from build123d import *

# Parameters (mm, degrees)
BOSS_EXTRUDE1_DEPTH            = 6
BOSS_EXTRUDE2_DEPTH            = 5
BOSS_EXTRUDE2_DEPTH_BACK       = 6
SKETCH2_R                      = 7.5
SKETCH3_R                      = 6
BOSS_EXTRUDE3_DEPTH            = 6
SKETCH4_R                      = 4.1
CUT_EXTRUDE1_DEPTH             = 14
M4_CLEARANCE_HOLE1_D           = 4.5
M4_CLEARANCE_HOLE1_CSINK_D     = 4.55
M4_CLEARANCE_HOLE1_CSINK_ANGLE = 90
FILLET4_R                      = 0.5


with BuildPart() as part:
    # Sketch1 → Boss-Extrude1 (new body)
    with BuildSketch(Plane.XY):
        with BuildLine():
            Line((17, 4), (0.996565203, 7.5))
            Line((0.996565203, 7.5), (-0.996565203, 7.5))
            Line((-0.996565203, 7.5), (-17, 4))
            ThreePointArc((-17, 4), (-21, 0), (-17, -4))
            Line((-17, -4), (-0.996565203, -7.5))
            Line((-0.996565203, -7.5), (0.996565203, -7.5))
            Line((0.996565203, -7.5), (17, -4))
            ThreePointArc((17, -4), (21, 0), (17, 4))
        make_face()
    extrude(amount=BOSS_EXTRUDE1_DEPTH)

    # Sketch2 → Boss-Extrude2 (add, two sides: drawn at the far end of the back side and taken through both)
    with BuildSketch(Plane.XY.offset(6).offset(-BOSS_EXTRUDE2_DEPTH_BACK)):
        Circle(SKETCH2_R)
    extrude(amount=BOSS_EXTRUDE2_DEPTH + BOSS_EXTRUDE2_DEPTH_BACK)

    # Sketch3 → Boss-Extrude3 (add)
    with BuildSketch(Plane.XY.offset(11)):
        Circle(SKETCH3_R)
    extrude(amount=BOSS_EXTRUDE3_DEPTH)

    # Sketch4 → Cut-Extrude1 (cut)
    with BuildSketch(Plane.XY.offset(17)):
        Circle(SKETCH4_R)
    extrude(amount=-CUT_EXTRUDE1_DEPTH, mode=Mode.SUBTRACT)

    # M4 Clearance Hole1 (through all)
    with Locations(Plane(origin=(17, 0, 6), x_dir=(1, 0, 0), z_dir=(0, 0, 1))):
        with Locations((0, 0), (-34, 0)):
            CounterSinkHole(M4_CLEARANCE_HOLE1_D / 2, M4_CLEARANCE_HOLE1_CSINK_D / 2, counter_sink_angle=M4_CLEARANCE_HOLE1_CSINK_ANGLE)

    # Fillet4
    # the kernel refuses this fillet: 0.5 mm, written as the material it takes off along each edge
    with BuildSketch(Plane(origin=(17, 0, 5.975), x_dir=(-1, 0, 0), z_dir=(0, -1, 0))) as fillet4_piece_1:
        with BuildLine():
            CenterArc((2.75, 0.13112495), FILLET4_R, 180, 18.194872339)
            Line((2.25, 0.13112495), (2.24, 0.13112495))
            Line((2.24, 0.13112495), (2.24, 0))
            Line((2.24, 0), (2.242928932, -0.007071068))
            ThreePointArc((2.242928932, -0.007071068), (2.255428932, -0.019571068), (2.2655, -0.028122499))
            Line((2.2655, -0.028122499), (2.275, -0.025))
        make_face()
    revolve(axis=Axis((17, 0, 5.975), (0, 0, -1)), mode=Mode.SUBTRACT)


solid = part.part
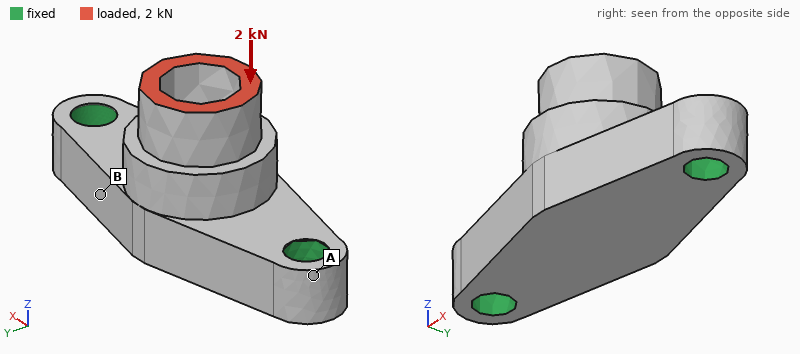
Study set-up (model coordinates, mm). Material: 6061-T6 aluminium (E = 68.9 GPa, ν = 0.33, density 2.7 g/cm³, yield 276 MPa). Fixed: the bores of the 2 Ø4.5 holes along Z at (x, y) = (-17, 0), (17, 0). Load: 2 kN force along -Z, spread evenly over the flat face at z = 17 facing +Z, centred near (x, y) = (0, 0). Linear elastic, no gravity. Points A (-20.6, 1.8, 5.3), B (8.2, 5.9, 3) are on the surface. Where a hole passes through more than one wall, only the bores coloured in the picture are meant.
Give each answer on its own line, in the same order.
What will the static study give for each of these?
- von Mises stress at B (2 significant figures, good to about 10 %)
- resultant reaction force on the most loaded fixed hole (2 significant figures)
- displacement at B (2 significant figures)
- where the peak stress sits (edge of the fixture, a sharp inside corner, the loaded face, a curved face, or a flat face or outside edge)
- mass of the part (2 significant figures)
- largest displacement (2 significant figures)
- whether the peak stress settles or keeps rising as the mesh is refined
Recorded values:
38 MPa
1.0 kN
14 µm
edge of the fixture
9.0 g
23 µm
keeps rising
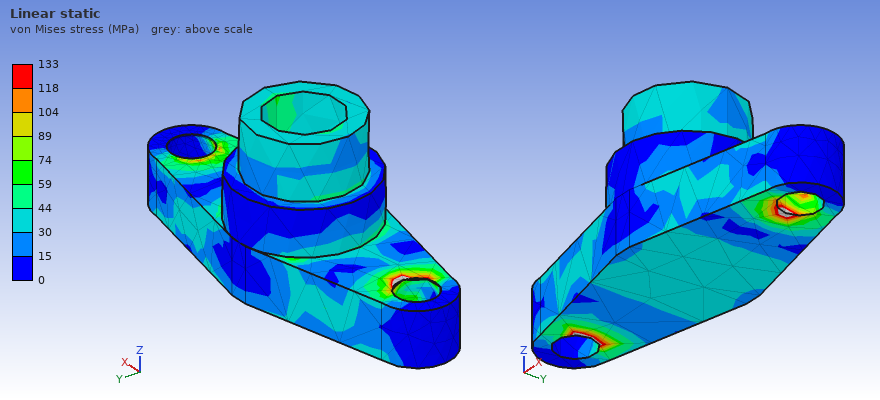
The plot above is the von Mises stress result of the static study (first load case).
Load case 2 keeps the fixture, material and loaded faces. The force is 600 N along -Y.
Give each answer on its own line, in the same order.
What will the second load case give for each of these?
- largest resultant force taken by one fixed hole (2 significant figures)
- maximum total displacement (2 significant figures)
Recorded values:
300 N
64 µm
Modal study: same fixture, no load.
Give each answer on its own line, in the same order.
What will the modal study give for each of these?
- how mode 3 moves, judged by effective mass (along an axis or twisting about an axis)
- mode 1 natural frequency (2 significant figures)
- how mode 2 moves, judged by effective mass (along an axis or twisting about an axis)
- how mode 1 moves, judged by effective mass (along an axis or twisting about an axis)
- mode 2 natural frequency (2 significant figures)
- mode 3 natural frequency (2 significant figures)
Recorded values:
along Y
14 kHz
along Z
along Y
21 kHz
30 kHz
